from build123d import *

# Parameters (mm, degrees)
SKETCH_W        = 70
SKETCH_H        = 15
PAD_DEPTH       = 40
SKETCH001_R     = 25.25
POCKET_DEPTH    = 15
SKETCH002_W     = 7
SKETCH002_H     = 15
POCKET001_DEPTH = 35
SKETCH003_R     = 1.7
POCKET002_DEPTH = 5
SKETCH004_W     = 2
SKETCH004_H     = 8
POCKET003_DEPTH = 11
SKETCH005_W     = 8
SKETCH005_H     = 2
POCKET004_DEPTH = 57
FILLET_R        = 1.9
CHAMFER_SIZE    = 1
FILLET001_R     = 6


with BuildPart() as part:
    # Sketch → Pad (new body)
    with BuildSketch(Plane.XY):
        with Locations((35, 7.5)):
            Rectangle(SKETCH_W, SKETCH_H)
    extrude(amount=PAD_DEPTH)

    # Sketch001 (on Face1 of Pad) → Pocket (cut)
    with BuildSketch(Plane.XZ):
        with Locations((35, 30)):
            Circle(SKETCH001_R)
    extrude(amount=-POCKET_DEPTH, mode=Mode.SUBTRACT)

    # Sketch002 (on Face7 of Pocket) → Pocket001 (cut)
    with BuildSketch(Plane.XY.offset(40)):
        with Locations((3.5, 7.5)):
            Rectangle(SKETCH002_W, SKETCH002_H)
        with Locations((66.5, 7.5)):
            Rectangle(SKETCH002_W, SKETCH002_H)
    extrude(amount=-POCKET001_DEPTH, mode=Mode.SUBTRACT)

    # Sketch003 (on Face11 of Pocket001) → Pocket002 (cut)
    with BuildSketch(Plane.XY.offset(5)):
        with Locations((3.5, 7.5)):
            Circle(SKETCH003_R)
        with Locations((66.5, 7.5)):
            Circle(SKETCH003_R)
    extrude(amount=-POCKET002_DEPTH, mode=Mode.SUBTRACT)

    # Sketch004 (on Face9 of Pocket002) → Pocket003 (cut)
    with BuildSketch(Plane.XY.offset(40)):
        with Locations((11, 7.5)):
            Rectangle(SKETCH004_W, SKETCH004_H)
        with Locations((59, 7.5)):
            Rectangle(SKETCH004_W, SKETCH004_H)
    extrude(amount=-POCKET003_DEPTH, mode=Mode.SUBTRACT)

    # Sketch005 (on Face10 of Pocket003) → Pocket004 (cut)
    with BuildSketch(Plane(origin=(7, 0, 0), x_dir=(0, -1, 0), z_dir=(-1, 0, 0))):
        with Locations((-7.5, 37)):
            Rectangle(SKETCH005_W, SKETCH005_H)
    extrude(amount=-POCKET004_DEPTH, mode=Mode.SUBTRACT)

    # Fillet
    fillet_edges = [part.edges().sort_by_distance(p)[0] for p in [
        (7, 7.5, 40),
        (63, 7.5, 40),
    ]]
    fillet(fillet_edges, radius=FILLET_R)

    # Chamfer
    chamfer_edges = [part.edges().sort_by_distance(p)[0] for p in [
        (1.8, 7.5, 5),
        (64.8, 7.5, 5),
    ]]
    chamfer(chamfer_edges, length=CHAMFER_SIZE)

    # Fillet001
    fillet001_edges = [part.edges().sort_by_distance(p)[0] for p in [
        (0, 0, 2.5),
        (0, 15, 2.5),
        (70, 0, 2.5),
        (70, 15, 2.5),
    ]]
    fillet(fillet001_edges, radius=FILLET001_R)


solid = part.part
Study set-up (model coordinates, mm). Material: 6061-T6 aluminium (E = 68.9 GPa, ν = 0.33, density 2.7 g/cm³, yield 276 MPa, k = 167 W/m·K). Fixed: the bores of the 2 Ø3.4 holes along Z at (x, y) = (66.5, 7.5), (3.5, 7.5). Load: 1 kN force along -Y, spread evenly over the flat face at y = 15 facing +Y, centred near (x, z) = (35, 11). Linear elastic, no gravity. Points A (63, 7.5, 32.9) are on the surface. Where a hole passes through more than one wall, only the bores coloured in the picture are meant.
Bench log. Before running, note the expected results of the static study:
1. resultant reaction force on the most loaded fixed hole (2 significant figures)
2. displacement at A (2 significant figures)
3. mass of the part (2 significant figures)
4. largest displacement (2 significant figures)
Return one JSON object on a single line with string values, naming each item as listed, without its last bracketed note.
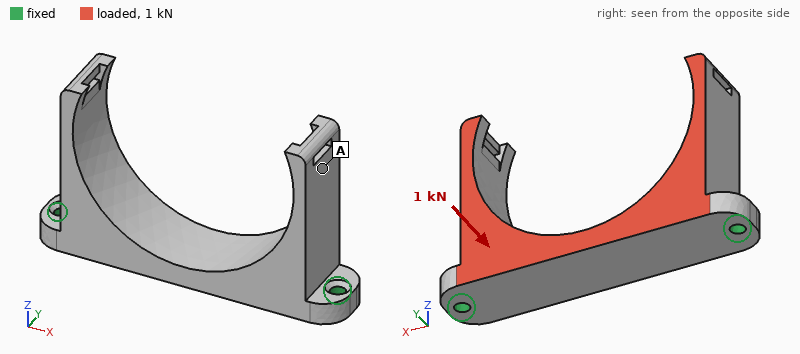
{"resultant reaction force on the most loaded fixed hole": "500 N", "displacement at A": "69 µm", "mass of the part": "32 g", "largest displacement": "91 µm"}
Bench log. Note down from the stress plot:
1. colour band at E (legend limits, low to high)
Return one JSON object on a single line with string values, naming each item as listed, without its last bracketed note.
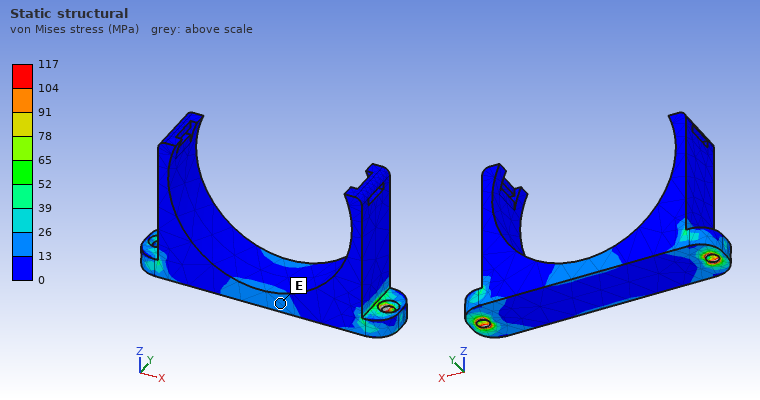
{"colour band at E": "13 to 26 MPa"}
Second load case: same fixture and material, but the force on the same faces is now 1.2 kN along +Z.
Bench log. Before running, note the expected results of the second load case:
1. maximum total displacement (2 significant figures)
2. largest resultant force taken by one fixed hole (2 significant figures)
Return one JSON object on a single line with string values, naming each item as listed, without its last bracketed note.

{"maximum total displacement": "0.12 mm", "largest resultant force taken by one fixed hole": "630 N"}
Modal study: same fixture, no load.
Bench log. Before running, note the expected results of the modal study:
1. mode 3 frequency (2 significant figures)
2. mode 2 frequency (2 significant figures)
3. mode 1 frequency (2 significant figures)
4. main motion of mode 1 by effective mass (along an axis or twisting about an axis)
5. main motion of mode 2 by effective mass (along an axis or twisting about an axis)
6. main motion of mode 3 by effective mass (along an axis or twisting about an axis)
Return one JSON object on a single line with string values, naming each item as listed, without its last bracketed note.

{"mode 3 frequency": "5300 Hz", "mode 2 frequency": "4200 Hz", "mode 1 frequency": "3400 Hz", "main motion of mode 1 by effective mass": "along Z", "main motion of mode 2 by effective mass": "along Y", "main motion of mode 3 by effective mass": "twisting about Z"}
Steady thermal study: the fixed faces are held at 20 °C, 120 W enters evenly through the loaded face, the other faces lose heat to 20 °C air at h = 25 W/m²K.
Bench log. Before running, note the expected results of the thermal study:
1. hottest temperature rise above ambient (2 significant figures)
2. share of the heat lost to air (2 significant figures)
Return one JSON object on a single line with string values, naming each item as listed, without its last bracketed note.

{"hottest temperature rise above ambient": "68 K", "share of the heat lost to air": "4.4 %"}
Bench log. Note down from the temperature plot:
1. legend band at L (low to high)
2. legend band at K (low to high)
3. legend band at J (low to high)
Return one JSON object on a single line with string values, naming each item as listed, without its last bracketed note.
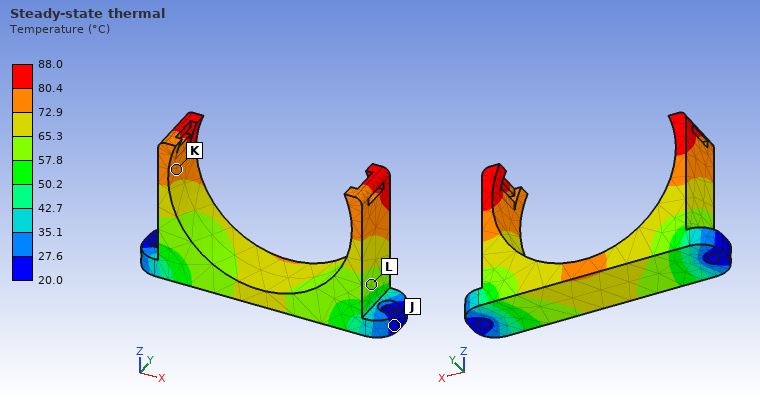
{"legend band at L": "57.8 to 65.3 °C", "legend band at K": "72.9 to 80.4 °C", "legend band at J": "20.0 to 27.6 °C"}
